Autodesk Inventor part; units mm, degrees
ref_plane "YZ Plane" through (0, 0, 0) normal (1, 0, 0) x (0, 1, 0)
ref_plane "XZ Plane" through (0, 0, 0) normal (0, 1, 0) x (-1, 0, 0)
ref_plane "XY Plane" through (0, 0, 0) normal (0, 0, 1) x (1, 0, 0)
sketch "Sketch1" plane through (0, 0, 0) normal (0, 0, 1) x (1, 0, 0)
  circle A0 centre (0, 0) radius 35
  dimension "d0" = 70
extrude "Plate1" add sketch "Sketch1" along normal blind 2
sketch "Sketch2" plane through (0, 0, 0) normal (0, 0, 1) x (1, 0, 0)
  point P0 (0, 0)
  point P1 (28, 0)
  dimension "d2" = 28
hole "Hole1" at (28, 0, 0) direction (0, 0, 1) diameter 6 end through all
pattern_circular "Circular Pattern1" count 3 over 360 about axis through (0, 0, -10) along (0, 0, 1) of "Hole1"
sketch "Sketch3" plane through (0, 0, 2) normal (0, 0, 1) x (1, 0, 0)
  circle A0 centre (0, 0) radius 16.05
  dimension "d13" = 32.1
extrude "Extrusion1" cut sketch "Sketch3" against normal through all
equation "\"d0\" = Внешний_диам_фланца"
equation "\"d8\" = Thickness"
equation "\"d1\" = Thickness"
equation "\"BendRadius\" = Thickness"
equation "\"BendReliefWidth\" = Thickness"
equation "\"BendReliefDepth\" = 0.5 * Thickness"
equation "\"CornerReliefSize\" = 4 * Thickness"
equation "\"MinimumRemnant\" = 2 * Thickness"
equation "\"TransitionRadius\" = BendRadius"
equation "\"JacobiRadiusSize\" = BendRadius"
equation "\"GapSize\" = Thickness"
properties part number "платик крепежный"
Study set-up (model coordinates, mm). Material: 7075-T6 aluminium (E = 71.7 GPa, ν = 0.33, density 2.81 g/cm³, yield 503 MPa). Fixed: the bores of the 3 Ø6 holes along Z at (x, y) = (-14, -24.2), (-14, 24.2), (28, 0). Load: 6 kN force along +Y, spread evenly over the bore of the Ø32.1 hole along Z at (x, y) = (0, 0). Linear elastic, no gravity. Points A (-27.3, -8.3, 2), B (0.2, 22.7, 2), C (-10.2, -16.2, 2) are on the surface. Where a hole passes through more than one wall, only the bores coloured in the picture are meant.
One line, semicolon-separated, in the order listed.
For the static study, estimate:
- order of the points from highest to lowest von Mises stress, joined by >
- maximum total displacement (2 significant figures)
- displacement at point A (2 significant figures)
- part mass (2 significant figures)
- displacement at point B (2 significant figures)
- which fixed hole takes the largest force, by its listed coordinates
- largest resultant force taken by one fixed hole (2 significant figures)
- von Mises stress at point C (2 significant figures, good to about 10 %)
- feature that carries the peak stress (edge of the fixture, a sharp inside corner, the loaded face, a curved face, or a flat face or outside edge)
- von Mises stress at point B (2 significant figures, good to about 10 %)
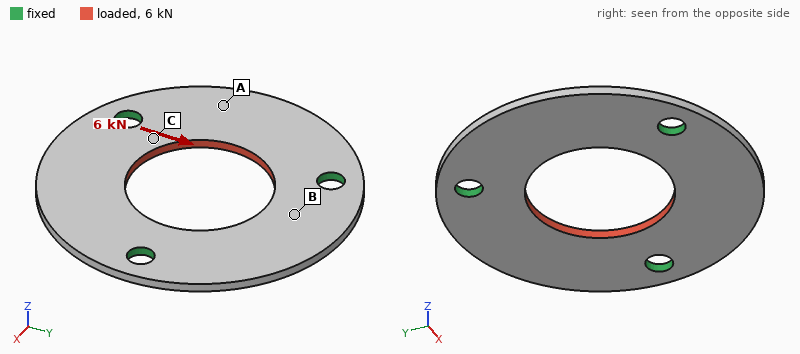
C > B > A; 24 µm; 5.8 µm; 17 g; 16 µm; (28, 0); 2.4 kN; 56 MPa; edge of the fixture; 35 MPa
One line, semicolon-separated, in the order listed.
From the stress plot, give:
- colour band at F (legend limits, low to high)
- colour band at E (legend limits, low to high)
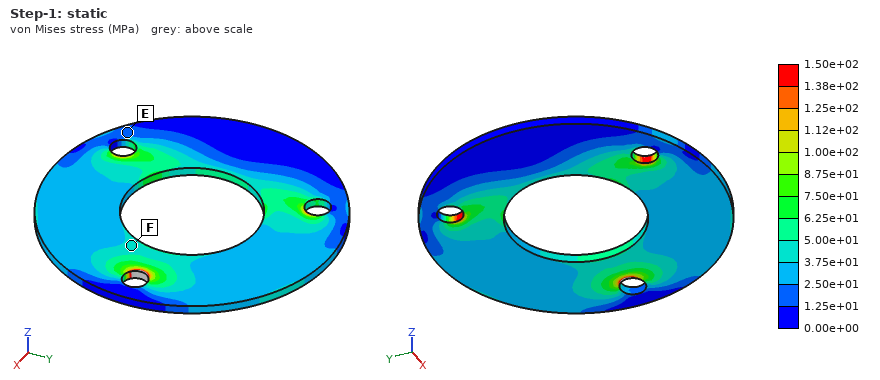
3.75e+01 to 5.00e+01 MPa; 1.25e+01 to 2.50e+01 MPa
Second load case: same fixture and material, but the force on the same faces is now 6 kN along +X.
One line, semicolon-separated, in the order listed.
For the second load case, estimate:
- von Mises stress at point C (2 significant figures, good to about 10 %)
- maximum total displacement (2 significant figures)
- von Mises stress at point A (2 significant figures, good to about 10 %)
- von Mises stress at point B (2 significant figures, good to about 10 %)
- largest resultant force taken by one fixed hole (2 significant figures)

47 MPa; 26 µm; 35 MPa; 31 MPa; 2.2 kN
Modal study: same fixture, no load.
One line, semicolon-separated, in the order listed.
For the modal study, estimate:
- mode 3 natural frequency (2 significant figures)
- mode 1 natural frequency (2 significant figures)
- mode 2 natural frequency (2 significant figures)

3300 Hz; 3200 Hz; 3200 Hz
